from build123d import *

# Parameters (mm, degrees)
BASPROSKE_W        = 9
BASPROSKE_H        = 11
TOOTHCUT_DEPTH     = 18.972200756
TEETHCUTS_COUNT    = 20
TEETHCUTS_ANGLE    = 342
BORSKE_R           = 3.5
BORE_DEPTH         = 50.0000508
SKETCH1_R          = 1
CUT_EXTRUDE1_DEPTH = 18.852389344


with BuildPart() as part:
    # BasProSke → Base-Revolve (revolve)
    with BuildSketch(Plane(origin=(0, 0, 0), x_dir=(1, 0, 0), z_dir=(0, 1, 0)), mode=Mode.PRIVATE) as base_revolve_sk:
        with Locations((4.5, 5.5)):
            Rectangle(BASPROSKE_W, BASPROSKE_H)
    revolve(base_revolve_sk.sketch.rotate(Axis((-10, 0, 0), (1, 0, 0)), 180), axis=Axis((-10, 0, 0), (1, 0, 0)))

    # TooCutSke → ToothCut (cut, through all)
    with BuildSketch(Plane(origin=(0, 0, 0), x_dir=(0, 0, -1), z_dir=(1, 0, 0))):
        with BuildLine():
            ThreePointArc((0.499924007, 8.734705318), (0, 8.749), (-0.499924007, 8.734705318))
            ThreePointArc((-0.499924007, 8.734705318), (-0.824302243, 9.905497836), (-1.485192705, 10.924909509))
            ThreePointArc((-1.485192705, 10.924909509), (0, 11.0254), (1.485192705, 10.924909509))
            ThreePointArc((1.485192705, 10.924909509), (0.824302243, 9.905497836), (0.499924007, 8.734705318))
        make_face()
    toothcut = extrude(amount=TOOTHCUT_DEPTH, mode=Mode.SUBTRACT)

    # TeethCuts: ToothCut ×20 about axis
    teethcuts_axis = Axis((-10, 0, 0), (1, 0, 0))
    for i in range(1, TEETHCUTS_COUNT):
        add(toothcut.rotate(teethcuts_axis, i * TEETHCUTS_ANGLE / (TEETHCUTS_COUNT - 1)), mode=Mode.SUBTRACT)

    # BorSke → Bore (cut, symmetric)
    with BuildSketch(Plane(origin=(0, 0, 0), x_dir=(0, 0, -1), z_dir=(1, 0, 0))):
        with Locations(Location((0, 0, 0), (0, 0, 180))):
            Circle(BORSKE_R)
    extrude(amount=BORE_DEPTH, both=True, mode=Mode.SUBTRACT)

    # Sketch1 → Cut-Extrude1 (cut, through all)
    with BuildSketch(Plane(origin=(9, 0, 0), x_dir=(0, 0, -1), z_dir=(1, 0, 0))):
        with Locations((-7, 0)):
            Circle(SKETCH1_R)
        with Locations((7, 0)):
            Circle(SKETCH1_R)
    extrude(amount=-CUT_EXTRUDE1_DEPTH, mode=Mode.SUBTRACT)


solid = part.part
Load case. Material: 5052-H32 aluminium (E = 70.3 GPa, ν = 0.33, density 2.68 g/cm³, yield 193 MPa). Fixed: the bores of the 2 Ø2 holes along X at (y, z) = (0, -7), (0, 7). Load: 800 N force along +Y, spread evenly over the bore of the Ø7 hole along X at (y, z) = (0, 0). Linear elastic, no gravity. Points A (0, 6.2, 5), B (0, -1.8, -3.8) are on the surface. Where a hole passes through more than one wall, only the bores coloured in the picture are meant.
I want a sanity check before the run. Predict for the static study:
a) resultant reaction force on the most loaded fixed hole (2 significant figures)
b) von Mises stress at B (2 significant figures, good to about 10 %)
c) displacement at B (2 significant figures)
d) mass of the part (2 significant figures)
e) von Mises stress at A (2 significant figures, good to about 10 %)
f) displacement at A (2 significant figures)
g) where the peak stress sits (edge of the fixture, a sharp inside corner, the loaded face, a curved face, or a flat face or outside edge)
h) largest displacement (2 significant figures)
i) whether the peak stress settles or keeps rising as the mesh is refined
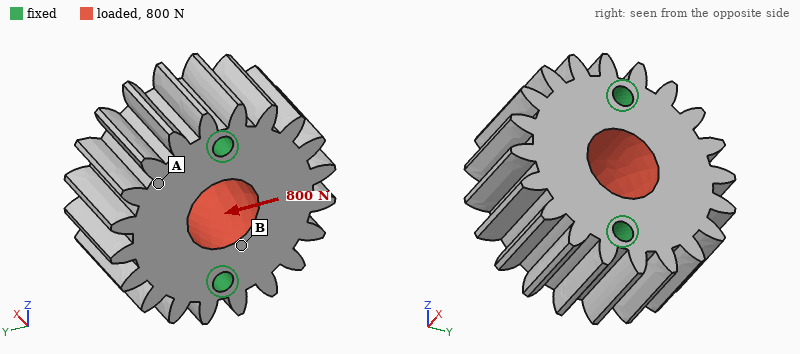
400 N
6.5 MPa
0.57 µm
6.2 g
3.3 MPa
0.48 µm
edge of the fixture
0.90 µm
keeps rising
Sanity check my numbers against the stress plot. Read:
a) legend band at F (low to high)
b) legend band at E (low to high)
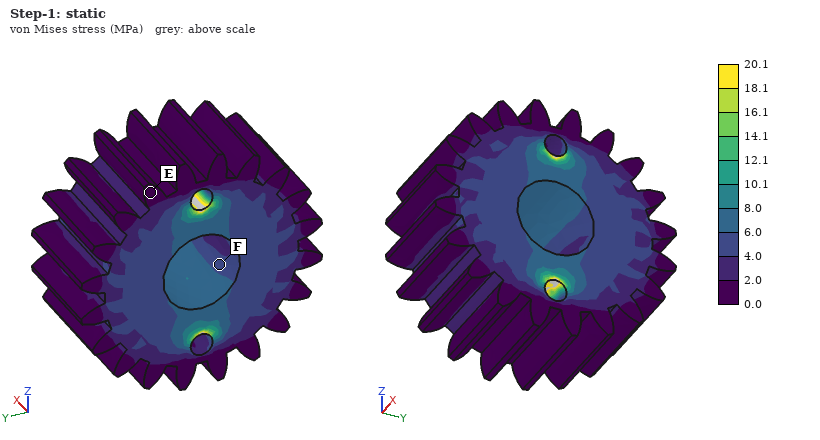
4.0 to 6.0 MPa
0.0 to 2.0 MPa
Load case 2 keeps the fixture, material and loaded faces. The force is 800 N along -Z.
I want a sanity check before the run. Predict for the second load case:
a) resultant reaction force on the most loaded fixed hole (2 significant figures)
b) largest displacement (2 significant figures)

400 N
0.80 µm
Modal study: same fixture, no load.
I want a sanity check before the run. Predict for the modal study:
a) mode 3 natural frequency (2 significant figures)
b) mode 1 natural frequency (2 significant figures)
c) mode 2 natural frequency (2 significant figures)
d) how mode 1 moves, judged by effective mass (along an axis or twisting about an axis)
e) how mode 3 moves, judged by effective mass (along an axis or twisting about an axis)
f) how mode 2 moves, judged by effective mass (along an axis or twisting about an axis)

64 kHz
44 kHz
49 kHz
twisting about Z
twisting about X
along X
